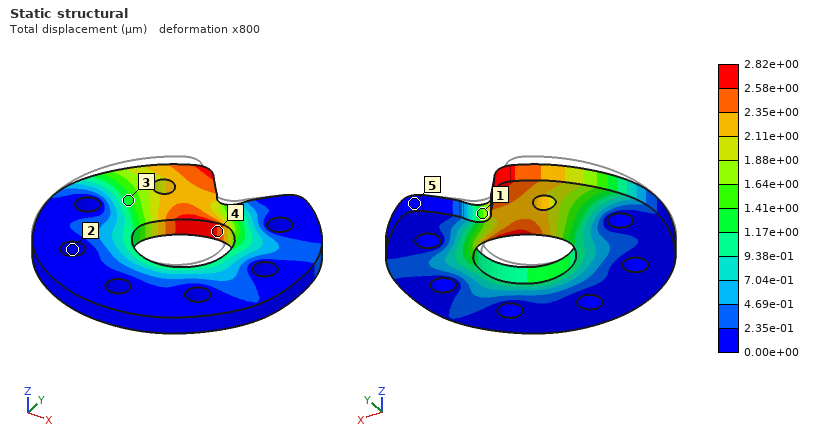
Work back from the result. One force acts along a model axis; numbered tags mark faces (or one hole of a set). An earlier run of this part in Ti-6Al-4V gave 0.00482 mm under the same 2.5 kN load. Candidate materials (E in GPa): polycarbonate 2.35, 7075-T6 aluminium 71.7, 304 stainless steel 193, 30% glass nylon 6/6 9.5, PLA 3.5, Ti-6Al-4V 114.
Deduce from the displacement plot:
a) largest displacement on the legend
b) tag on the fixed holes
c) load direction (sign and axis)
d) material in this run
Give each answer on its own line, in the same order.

2.82e+00 µm
2
+X
304 stainless steel
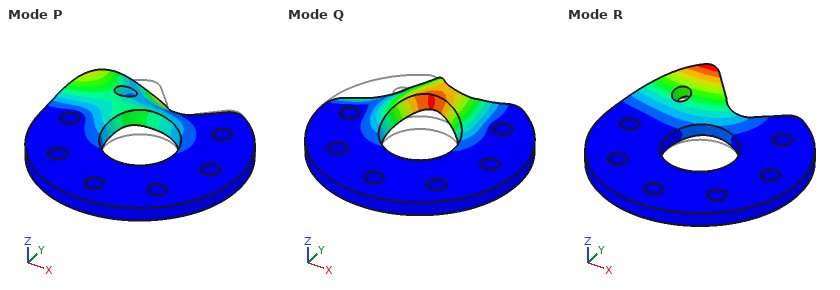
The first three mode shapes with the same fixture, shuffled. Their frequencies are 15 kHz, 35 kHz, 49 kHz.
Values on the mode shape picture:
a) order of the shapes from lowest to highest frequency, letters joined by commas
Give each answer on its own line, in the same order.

R, Q, P
